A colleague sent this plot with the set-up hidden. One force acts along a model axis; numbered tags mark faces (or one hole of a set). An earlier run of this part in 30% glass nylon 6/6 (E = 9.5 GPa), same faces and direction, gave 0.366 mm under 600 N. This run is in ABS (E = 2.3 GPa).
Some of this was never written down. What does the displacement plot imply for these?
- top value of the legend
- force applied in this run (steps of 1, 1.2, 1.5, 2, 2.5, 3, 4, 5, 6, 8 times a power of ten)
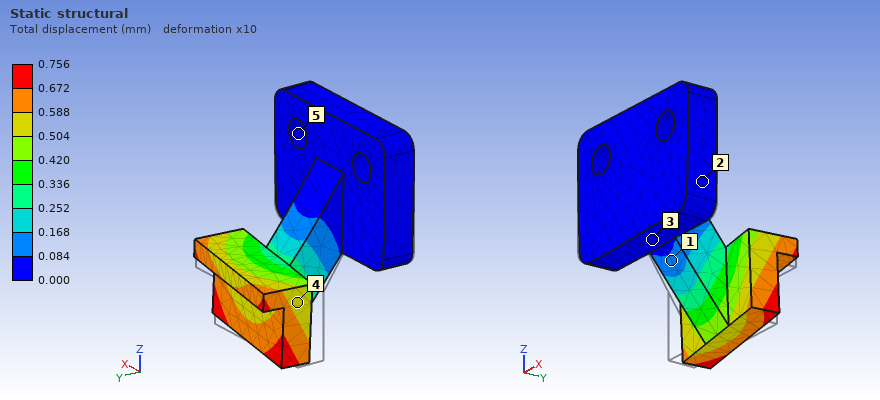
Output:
0.756 mm
300 N
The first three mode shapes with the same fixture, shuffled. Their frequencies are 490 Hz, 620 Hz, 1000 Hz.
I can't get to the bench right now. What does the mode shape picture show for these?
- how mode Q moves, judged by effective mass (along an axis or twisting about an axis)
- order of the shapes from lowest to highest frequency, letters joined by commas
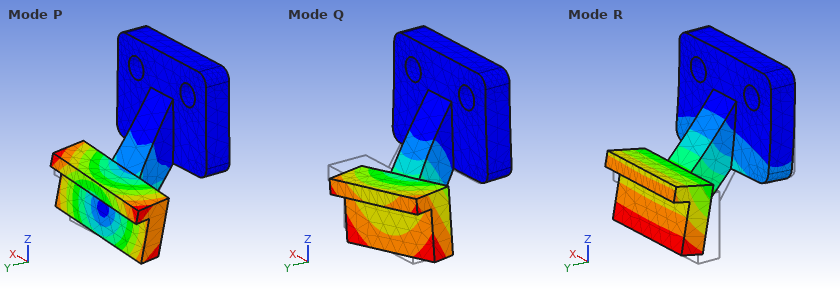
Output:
along X
R, Q, P
